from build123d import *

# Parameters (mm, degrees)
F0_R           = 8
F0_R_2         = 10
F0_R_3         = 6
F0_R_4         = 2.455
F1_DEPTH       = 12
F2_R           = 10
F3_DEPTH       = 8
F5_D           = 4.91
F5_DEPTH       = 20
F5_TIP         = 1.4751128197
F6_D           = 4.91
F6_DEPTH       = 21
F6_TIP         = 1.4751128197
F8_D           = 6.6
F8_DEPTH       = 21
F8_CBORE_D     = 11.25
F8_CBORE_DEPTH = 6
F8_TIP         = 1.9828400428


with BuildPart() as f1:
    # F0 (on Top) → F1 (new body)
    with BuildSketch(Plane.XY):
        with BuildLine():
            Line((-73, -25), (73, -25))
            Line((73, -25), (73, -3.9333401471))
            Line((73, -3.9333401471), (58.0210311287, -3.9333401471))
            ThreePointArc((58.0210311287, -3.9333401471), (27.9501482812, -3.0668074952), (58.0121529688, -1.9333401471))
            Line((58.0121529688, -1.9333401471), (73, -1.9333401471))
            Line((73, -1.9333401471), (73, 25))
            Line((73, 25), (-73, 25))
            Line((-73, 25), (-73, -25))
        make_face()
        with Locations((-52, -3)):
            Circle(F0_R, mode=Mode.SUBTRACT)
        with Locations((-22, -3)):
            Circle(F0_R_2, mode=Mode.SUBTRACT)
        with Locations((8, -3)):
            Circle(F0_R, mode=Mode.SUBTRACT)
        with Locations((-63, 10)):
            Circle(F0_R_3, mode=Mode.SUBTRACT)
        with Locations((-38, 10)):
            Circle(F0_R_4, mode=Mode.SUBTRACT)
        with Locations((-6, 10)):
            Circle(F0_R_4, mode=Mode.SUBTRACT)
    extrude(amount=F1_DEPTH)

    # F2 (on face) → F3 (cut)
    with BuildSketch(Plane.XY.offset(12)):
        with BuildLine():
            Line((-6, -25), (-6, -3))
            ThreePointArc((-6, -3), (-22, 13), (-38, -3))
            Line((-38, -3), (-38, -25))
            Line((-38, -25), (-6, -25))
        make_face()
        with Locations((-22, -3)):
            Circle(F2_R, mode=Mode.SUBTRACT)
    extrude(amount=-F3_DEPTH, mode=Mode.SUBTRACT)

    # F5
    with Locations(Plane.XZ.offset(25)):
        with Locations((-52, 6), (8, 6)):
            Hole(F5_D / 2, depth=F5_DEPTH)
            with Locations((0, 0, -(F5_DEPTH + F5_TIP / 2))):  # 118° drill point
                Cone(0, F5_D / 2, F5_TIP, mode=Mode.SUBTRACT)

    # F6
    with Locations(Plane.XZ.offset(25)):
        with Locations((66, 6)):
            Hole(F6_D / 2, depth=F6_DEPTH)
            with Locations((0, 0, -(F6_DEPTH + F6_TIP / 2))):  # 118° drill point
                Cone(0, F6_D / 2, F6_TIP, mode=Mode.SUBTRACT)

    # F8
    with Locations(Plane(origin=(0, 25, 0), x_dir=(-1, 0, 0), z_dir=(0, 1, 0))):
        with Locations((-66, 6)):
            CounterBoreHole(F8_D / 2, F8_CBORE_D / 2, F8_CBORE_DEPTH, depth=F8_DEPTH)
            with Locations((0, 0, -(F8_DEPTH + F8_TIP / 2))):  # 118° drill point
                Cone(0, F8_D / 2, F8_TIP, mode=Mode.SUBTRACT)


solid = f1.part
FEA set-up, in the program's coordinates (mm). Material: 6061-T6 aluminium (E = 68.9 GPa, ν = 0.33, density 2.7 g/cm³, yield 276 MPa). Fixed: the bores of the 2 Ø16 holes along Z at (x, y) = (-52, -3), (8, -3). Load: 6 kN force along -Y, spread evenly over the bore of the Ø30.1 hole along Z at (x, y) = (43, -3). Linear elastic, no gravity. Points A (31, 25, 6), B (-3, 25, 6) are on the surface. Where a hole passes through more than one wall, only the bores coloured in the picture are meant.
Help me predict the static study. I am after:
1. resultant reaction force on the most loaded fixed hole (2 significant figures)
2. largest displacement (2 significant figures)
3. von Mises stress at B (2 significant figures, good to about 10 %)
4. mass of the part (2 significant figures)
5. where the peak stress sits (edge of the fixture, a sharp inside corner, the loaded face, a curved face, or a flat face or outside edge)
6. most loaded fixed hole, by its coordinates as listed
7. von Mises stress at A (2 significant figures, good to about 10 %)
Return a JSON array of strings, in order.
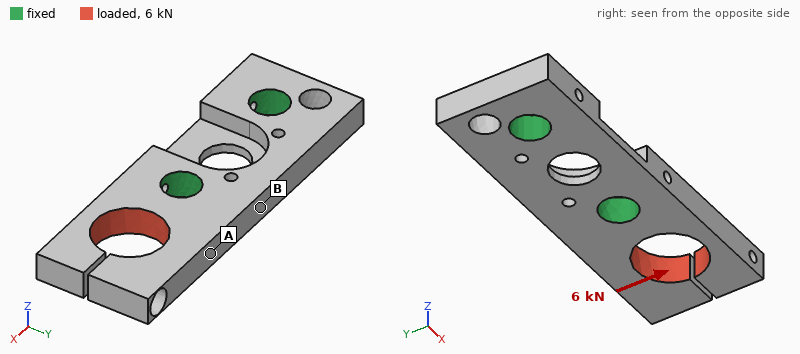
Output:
["6.9 kN", "0.56 mm", "25 MPa", "160 g", "the loaded face", "(8, -3)", "56 MPa"]
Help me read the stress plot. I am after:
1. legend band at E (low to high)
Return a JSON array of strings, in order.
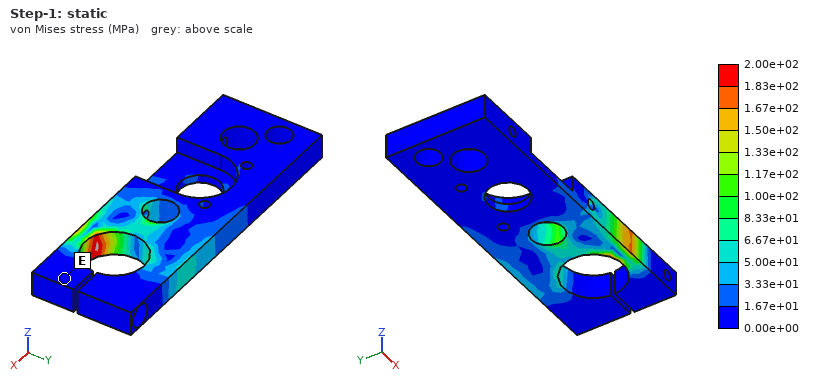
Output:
["0.00e+00 to 1.67e+01 MPa"]
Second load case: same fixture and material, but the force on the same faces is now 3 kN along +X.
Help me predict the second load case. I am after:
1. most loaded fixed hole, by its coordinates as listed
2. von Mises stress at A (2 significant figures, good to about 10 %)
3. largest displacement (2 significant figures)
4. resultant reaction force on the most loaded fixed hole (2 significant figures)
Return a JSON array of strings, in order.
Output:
["(8, -3)", "11 MPa", "0.16 mm", "2.8 kN"]
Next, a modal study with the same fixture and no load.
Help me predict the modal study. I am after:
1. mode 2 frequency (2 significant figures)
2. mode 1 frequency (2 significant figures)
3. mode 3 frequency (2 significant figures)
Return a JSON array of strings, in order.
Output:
["2300 Hz", "2100 Hz", "2500 Hz"]
